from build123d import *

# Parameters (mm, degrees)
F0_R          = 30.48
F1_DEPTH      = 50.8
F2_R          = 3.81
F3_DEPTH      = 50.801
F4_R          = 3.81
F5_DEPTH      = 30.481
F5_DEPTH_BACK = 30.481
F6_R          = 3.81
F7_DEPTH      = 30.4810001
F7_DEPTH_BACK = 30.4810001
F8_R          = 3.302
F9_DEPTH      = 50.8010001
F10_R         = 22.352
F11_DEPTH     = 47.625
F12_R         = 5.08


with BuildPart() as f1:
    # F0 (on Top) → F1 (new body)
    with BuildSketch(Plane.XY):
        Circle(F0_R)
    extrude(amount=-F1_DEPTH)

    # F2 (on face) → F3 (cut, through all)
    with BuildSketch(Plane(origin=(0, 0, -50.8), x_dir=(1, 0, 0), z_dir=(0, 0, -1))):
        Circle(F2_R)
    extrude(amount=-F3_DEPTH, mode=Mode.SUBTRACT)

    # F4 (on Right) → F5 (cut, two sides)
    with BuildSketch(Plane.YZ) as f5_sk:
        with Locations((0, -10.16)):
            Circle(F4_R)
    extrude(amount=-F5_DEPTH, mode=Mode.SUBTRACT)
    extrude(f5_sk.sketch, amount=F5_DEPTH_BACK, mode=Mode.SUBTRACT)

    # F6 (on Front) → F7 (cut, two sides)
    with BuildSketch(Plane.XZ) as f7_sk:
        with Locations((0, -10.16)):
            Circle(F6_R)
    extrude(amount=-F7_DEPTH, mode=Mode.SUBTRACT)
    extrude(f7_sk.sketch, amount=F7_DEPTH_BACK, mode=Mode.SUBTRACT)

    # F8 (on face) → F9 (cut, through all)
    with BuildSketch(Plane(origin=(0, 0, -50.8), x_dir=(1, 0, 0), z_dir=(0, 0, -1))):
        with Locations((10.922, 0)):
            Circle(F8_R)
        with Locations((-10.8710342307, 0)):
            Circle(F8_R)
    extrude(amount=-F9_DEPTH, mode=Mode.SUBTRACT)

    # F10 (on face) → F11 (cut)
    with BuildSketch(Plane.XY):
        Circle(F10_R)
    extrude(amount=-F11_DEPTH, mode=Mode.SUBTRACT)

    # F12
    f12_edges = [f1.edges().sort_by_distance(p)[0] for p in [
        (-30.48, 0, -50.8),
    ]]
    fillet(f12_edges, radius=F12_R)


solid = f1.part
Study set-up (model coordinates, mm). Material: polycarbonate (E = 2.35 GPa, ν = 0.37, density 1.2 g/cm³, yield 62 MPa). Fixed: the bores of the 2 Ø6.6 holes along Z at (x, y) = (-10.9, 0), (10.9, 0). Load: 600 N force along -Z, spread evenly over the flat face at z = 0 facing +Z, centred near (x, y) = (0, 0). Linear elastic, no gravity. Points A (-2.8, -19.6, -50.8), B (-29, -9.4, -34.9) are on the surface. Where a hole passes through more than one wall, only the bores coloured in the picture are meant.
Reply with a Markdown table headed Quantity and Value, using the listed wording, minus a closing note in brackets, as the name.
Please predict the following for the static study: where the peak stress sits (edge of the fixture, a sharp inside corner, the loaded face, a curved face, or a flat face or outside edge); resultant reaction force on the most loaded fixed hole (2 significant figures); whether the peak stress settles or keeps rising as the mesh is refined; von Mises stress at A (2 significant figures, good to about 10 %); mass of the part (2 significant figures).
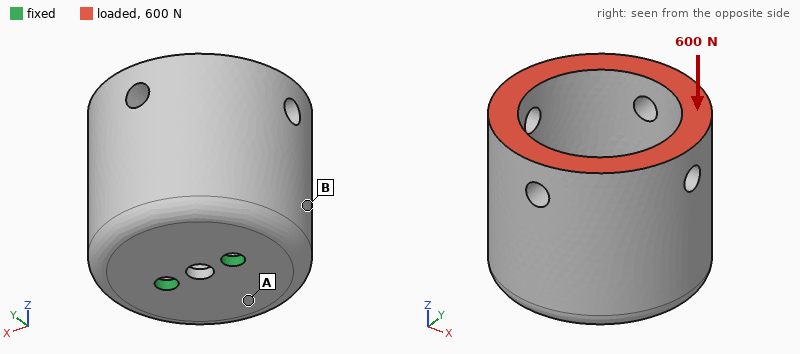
| Quantity | Value |
|---|---|
| where the peak stress sits | edge of the fixture |
| resultant reaction force on the most loaded fixed hole | 310 N |
| whether the peak stress settles or keeps rising as the mesh is refined | keeps rising |
| von Mises stress at A | 4.9 MPa |
| mass of the part | 85 g |
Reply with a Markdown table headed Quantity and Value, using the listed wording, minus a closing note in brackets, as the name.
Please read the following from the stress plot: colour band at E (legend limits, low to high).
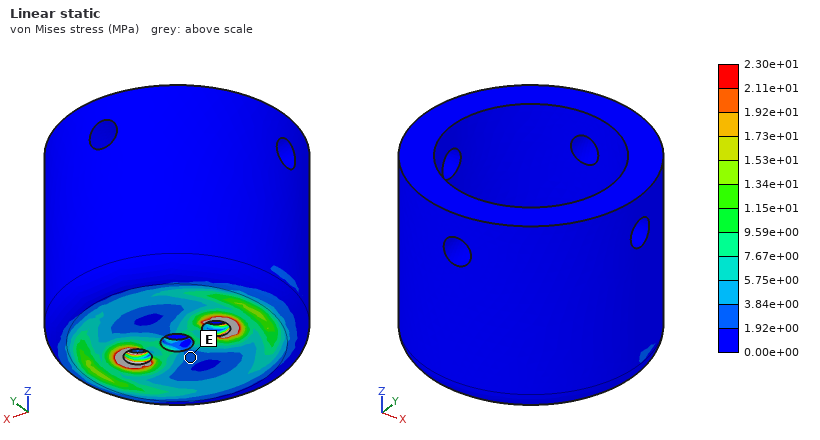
| Quantity | Value |
|---|---|
| colour band at E | 1.92e+00 to 3.84e+00 MPa |
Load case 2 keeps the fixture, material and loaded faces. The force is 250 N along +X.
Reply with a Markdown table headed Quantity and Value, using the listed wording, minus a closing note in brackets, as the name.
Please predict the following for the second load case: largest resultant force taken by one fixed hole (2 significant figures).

| Quantity | Value |
|---|---|
| largest resultant force taken by one fixed hole | 390 N |
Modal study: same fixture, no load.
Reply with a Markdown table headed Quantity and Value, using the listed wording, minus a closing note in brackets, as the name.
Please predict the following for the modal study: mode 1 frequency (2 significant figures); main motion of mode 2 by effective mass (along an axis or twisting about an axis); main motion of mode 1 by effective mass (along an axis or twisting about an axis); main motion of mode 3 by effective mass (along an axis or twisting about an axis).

| Quantity | Value |
|---|---|
| mode 1 frequency | 210 Hz |
| main motion of mode 2 by effective mass | along X |
| main motion of mode 1 by effective mass | along Y |
| main motion of mode 3 by effective mass | along Z |
